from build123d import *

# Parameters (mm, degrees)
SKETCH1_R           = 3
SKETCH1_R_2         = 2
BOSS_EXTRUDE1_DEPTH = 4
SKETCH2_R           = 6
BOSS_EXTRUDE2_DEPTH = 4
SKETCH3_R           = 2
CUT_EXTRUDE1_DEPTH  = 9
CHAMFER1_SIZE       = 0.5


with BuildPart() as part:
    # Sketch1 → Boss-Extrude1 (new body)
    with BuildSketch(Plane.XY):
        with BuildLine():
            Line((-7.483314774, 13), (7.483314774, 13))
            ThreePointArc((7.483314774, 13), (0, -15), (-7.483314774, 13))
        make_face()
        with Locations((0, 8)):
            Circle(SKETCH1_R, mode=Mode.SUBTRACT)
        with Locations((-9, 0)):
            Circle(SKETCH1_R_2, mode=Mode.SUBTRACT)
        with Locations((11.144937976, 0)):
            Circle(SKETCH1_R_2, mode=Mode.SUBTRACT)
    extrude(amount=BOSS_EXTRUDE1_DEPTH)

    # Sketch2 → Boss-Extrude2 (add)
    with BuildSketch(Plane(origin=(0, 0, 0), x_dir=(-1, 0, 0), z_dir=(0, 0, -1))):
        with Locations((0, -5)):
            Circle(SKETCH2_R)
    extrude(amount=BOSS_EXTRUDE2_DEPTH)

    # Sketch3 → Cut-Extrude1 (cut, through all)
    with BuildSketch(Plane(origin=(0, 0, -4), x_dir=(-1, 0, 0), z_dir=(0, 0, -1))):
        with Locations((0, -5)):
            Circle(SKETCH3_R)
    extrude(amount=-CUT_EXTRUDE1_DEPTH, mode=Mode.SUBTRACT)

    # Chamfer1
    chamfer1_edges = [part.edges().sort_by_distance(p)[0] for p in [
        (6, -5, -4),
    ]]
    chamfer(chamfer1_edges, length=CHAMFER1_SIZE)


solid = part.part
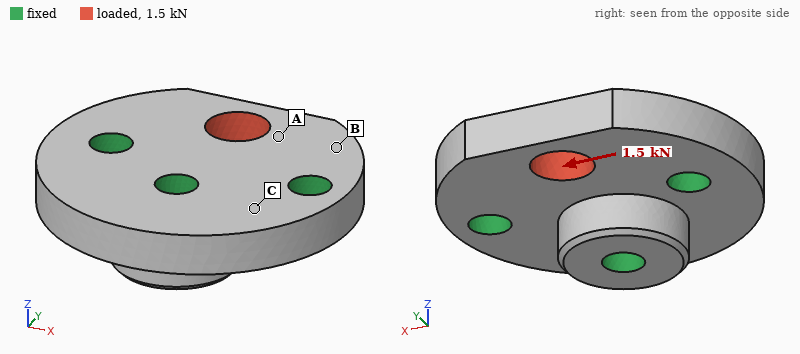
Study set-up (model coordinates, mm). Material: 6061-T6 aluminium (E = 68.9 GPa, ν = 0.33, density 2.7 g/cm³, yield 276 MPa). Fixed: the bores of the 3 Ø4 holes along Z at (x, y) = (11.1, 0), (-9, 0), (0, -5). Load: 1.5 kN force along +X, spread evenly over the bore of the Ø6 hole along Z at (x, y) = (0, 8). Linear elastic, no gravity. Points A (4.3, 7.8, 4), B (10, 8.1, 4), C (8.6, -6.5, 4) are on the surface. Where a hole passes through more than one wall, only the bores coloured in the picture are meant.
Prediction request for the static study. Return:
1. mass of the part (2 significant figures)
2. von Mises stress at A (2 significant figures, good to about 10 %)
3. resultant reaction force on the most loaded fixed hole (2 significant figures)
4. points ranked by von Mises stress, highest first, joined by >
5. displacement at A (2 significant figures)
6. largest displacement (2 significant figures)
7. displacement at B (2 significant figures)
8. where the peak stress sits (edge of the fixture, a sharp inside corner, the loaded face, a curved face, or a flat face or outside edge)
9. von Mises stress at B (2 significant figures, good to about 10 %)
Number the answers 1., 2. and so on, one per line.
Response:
1. 7.8 g
2. 34 MPa
3. 850 N
4. A > B > C
5. 5.3 µm
6. 9.1 µm
7. 4.6 µm
8. edge of the fixture
9. 16 MPa
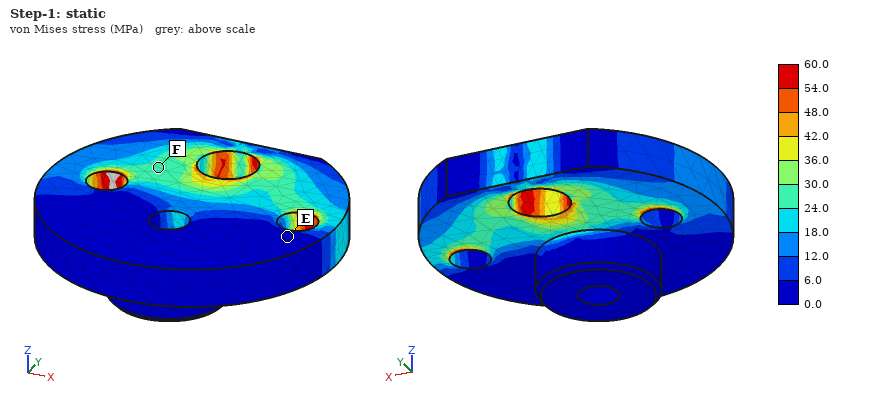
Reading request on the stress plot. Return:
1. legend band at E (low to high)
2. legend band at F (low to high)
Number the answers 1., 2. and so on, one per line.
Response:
1. 0.0 to 6.0 MPa
2. 24.0 to 30.0 MPa
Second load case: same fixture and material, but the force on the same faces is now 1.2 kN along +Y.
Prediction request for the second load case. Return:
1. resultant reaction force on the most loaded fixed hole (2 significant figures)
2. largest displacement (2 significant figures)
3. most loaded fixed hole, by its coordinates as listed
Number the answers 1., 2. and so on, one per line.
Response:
1. 520 N
2. 6.5 µm
3. (0, -5)
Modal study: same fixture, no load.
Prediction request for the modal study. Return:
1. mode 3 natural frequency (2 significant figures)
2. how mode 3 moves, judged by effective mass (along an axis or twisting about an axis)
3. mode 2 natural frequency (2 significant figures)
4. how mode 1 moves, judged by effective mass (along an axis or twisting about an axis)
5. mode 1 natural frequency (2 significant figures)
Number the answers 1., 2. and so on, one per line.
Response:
1. 52 kHz
2. along Z
3. 36 kHz
4. along Z
5. 22 kHz
